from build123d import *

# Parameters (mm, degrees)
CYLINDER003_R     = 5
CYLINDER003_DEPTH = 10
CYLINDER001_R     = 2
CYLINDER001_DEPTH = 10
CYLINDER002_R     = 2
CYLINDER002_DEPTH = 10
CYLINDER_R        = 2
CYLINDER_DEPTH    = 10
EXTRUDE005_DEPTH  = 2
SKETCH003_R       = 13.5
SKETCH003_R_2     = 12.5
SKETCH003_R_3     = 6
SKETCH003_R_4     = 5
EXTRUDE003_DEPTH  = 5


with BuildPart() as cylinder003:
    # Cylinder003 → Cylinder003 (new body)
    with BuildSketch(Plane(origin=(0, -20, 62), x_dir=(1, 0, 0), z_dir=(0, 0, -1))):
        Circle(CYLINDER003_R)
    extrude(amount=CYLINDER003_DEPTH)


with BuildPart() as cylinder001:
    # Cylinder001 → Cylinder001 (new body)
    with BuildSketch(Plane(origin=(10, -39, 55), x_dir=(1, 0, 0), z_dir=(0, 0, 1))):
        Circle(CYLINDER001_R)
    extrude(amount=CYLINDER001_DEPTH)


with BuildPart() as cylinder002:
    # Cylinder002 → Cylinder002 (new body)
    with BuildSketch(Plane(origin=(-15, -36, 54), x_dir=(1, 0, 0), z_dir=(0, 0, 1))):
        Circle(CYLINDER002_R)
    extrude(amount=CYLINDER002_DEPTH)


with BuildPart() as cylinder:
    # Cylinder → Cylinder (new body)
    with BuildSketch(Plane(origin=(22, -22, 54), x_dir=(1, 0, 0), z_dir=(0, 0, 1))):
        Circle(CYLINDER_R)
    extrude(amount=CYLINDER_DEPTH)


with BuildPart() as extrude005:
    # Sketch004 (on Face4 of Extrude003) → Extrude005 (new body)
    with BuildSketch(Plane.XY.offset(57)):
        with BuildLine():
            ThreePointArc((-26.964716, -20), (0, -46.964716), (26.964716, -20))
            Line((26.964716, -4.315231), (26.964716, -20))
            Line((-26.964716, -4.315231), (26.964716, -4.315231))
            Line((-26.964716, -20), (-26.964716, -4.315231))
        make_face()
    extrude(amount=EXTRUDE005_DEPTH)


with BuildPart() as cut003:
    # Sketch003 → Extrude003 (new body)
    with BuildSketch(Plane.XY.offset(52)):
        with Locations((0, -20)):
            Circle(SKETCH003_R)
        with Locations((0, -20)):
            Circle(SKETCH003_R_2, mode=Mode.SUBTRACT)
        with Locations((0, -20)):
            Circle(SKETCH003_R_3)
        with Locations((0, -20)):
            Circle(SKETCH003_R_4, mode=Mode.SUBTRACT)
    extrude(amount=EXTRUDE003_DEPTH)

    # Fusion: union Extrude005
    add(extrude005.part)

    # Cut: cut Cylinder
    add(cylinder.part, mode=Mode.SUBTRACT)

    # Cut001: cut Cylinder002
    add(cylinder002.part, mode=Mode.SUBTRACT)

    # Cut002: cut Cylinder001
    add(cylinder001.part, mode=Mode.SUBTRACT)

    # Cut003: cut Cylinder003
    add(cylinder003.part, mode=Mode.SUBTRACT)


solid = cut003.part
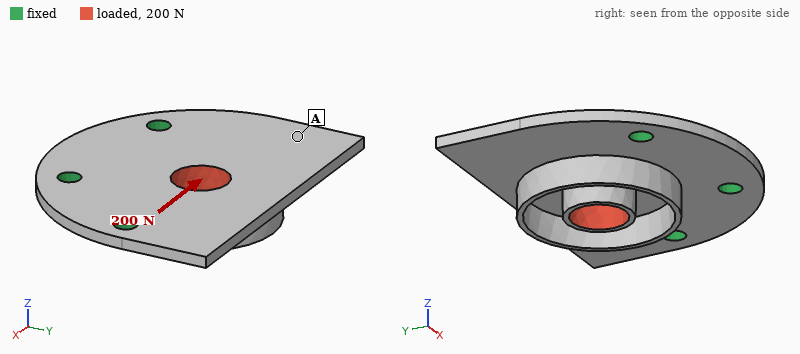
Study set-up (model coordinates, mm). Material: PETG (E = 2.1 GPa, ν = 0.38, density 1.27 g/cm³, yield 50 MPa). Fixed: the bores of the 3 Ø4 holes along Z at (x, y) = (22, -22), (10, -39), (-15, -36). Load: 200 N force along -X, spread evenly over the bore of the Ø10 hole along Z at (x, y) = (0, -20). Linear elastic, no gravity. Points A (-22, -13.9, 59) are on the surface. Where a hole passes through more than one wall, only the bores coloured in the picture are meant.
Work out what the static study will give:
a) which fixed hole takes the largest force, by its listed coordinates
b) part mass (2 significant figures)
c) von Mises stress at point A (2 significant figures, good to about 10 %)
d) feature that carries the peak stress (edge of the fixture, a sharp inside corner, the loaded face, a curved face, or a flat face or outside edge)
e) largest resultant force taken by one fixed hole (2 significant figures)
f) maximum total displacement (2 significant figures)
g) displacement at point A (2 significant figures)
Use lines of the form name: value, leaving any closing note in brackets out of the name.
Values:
which fixed hole takes the largest force, by its listed coordinates: (22, -22)
part mass: 5.5 g
von Mises stress at point A: 2.0 MPa
feature that carries the peak stress: a flat face or outside edge
largest resultant force taken by one fixed hole: 110 N
maximum total displacement: 0.71 mm
displacement at point A: 0.46 mm
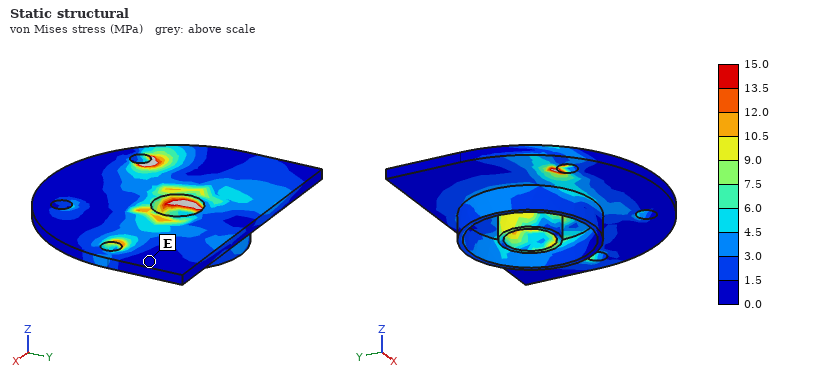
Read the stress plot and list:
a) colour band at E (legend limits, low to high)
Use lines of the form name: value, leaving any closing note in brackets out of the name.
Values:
colour band at E: 0.0 to 1.5 MPa
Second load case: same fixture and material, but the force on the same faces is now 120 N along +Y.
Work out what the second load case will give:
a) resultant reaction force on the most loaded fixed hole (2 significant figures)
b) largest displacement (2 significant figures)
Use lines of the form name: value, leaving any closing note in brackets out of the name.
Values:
resultant reaction force on the most loaded fixed hole: 56 N
largest displacement: 0.74 mm
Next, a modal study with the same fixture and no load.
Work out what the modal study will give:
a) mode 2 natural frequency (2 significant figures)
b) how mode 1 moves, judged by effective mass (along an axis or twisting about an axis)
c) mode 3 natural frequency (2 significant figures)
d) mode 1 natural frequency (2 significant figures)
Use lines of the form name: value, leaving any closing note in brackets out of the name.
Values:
mode 2 natural frequency: 1300 Hz
how mode 1 moves, judged by effective mass: along Z
mode 3 natural frequency: 2200 Hz
mode 1 natural frequency: 560 Hz
